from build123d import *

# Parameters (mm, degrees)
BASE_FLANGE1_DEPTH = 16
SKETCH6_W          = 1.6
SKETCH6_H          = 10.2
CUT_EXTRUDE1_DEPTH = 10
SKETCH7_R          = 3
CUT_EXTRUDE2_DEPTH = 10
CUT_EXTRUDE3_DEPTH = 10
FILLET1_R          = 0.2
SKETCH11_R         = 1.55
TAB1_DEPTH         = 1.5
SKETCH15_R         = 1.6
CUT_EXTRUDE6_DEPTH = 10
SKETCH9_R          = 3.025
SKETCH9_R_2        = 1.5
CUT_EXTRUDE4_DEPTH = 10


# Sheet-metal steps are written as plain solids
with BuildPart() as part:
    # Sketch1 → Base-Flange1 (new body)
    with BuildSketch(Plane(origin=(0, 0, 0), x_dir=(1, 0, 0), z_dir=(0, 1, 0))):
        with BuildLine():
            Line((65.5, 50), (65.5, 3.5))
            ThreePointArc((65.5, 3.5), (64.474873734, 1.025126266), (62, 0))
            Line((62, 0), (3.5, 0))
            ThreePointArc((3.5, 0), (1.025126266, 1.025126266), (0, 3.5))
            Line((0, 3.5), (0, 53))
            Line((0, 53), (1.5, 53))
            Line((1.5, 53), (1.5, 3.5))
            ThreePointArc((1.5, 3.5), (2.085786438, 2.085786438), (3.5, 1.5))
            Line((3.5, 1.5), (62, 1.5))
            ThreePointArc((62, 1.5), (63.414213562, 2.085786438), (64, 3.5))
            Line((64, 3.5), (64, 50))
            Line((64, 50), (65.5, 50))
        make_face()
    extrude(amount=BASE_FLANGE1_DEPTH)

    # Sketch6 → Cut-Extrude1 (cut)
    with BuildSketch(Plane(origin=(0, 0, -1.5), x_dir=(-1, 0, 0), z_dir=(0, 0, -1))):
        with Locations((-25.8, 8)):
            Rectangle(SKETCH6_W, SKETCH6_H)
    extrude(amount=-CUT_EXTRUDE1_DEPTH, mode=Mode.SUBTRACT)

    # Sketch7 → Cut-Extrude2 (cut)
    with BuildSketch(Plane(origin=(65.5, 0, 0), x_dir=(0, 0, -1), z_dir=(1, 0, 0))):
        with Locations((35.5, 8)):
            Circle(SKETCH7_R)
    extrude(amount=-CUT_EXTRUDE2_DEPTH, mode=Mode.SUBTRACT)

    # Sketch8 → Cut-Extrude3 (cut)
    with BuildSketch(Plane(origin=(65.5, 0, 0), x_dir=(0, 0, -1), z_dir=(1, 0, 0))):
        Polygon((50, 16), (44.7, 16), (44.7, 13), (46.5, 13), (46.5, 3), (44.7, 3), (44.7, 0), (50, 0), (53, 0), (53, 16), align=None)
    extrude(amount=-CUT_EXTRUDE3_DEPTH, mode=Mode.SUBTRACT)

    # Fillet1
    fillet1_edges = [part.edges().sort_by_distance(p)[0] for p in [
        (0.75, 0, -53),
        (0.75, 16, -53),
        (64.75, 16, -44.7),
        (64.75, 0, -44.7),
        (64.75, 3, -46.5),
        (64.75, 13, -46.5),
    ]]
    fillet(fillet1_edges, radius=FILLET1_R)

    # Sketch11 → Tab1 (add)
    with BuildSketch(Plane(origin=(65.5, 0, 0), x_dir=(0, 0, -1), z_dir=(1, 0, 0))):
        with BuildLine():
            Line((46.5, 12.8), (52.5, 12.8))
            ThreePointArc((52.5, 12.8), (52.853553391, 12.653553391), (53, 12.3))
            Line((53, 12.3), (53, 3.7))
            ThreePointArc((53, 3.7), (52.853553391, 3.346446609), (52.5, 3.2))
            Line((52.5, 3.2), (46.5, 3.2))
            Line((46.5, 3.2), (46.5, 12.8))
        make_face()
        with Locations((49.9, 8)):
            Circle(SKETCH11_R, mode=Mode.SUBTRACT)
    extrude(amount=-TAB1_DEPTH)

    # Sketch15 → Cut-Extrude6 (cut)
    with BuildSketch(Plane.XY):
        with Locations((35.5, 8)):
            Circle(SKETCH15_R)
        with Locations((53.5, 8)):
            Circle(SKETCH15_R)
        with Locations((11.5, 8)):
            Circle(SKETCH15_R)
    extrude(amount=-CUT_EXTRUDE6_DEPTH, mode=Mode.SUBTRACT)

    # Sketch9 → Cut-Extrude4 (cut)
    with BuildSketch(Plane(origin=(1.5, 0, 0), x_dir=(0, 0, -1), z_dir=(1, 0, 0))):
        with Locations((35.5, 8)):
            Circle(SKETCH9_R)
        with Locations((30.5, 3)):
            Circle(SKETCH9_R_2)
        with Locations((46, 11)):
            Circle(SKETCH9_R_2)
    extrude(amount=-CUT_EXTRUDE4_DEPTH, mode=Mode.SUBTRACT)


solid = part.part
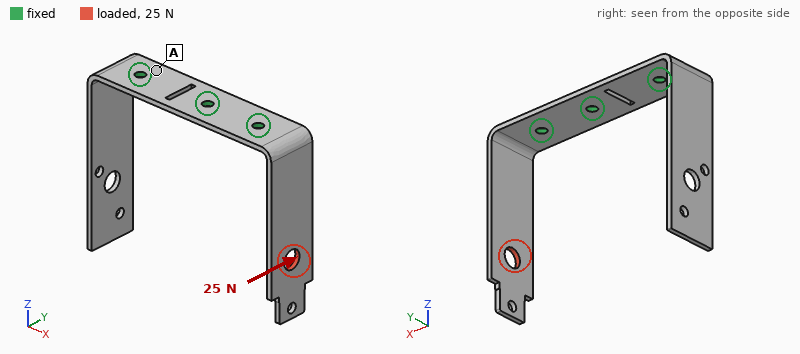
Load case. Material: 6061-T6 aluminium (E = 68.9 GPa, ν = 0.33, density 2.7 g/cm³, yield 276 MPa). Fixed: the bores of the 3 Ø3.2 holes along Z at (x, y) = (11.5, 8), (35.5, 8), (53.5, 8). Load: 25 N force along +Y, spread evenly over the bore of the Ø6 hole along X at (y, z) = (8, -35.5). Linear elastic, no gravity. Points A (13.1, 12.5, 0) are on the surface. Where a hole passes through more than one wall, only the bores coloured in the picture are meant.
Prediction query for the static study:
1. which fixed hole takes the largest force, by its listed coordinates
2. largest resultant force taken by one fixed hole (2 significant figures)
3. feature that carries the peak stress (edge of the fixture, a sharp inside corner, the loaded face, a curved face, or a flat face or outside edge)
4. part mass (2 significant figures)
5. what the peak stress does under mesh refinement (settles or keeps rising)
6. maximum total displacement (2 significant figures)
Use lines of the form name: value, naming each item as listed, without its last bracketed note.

which fixed hole takes the largest force, by its listed coordinates: (53.5, 8)
largest resultant force taken by one fixed hole: 36 N
feature that carries the peak stress: edge of the fixture
part mass: 10 g
what the peak stress does under mesh refinement: keeps rising
maximum total displacement: 0.86 mm
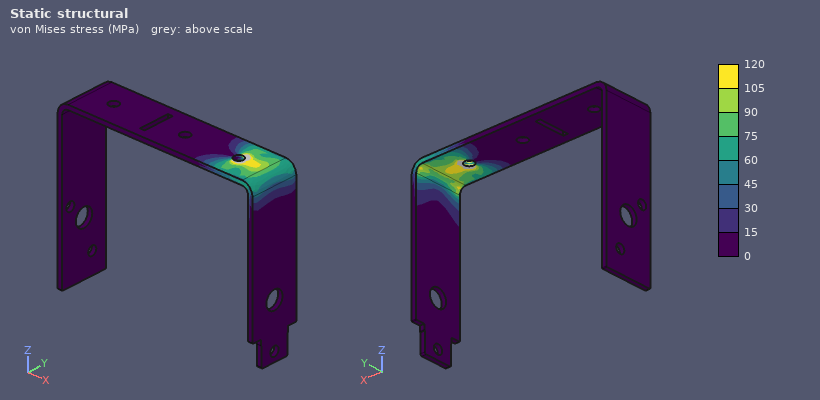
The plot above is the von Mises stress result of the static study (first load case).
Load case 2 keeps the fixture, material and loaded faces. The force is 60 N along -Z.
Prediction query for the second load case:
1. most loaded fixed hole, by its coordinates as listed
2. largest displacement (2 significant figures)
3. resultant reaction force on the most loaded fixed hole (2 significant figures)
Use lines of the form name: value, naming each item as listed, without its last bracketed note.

most loaded fixed hole, by its coordinates as listed: (53.5, 8)
largest displacement: 0.58 mm
resultant reaction force on the most loaded fixed hole: 65 N
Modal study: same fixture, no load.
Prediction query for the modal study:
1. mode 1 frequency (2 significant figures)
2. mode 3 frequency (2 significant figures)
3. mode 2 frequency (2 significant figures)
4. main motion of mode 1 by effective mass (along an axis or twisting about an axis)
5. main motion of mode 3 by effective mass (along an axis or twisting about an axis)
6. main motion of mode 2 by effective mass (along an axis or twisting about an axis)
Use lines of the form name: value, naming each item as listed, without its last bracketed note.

mode 1 frequency: 360 Hz
mode 3 frequency: 700 Hz
mode 2 frequency: 400 Hz
main motion of mode 1 by effective mass: along X
main motion of mode 3 by effective mass: along Y
main motion of mode 2 by effective mass: along X
